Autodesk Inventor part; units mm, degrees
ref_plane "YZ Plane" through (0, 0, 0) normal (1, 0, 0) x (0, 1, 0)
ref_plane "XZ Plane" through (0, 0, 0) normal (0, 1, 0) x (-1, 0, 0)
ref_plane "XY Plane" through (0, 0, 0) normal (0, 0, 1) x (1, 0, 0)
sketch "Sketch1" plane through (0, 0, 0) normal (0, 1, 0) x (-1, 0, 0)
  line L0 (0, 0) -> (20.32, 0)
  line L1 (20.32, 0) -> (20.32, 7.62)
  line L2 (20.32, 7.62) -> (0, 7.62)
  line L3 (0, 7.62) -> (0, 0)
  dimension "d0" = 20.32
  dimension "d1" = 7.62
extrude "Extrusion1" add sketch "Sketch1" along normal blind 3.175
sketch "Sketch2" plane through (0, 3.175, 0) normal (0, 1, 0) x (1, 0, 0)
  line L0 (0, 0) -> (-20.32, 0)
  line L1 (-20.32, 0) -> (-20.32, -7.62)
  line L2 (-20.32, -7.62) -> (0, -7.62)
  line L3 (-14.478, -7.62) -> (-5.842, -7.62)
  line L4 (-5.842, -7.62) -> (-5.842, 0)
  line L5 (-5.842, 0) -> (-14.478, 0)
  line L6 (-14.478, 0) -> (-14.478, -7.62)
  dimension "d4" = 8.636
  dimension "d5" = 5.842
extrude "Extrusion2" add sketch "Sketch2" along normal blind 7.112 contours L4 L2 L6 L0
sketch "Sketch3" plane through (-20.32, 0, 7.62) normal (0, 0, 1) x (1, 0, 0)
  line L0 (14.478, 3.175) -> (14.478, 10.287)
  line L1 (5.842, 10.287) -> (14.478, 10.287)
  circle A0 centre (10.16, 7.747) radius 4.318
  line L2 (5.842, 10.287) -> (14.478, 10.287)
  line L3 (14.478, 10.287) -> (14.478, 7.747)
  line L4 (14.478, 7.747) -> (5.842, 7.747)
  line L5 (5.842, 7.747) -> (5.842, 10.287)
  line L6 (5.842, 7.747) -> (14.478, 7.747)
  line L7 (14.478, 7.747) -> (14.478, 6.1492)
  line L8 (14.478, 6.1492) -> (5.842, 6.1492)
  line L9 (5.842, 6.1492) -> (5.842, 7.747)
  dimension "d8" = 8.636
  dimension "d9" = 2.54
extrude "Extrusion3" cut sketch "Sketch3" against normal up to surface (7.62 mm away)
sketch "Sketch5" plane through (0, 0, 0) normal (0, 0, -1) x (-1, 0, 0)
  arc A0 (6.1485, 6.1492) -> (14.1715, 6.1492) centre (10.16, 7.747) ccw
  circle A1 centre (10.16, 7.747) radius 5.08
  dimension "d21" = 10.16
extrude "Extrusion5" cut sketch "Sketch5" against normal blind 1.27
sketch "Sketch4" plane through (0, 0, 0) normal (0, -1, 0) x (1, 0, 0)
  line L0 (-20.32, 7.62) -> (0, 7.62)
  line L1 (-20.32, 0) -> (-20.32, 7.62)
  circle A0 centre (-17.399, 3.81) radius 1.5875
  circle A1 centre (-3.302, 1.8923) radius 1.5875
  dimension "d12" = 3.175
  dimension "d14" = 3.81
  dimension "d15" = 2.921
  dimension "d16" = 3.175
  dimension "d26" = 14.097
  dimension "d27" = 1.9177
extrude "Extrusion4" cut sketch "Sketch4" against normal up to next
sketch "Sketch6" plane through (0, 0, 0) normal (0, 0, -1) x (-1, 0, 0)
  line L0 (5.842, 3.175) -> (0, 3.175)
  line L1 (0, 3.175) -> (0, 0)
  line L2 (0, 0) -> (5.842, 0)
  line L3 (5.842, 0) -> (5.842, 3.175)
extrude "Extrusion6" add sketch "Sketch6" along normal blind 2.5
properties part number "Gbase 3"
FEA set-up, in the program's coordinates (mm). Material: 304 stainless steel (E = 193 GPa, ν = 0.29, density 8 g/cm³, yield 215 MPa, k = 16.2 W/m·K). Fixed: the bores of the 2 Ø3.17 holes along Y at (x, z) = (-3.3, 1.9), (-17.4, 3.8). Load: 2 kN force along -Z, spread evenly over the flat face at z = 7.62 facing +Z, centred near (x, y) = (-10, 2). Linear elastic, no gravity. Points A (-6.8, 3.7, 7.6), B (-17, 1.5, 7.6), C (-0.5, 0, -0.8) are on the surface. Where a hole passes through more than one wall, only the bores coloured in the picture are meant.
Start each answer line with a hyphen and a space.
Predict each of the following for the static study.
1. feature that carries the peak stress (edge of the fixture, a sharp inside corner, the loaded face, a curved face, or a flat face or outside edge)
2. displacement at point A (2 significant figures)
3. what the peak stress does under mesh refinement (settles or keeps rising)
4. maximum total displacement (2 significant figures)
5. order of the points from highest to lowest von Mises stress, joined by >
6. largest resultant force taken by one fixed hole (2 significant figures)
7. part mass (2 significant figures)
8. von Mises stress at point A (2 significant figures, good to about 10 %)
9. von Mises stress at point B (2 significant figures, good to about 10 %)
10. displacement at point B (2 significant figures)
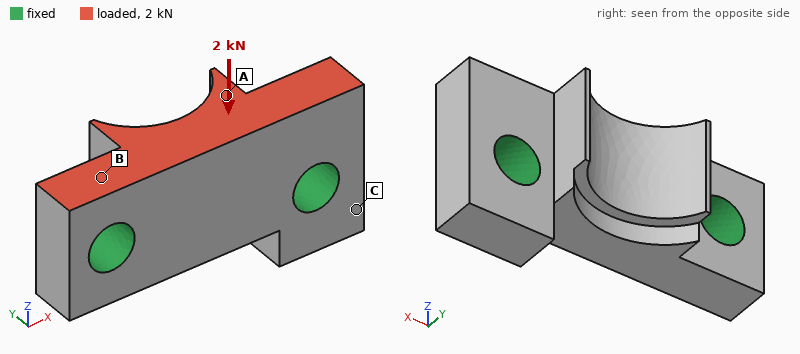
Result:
- edge of the fixture
- 2.3 µm
- keeps rising
- 2.8 µm
- B > A > C
- 1.1 kN
- 4.4 g
- 26 MPa
- 47 MPa
- 0.58 µm
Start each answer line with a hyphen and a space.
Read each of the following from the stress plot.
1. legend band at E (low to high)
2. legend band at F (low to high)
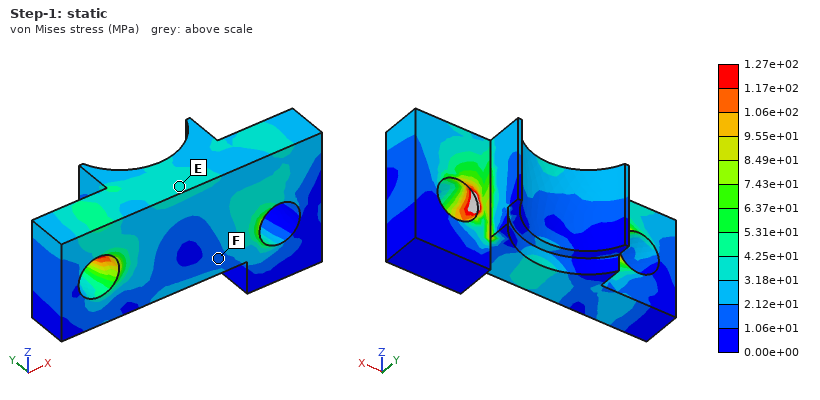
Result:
- 3.18e+01 to 4.25e+01 MPa
- 1.06e+01 to 2.12e+01 MPa
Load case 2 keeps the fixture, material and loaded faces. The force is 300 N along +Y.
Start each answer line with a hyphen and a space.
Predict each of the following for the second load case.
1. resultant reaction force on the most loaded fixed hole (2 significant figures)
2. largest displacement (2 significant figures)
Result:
- 160 N
- 2.4 µm
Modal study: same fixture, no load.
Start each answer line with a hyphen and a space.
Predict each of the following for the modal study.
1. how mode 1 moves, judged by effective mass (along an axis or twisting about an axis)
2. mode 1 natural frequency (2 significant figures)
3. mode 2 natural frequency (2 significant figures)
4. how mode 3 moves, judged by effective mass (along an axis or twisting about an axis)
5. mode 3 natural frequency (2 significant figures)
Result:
- along Y
- 60 kHz
- 79 kHz
- along Z
- 87 kHz
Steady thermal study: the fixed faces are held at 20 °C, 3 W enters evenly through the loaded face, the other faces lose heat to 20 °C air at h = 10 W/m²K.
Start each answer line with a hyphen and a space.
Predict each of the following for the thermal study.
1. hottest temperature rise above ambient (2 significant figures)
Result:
- 17 K
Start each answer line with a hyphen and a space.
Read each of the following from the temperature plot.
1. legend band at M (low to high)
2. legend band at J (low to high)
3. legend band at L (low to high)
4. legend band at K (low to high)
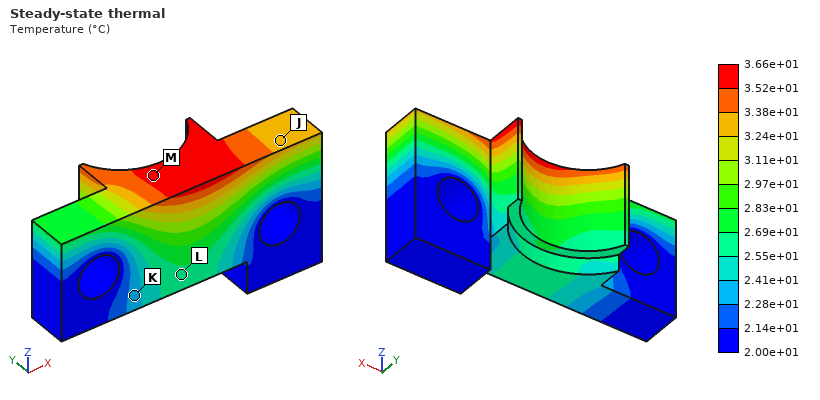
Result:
- 3.52e+01 to 3.66e+01 °C
- 3.24e+01 to 3.38e+01 °C
- 2.55e+01 to 2.69e+01 °C
- 2.28e+01 to 2.41e+01 °C
